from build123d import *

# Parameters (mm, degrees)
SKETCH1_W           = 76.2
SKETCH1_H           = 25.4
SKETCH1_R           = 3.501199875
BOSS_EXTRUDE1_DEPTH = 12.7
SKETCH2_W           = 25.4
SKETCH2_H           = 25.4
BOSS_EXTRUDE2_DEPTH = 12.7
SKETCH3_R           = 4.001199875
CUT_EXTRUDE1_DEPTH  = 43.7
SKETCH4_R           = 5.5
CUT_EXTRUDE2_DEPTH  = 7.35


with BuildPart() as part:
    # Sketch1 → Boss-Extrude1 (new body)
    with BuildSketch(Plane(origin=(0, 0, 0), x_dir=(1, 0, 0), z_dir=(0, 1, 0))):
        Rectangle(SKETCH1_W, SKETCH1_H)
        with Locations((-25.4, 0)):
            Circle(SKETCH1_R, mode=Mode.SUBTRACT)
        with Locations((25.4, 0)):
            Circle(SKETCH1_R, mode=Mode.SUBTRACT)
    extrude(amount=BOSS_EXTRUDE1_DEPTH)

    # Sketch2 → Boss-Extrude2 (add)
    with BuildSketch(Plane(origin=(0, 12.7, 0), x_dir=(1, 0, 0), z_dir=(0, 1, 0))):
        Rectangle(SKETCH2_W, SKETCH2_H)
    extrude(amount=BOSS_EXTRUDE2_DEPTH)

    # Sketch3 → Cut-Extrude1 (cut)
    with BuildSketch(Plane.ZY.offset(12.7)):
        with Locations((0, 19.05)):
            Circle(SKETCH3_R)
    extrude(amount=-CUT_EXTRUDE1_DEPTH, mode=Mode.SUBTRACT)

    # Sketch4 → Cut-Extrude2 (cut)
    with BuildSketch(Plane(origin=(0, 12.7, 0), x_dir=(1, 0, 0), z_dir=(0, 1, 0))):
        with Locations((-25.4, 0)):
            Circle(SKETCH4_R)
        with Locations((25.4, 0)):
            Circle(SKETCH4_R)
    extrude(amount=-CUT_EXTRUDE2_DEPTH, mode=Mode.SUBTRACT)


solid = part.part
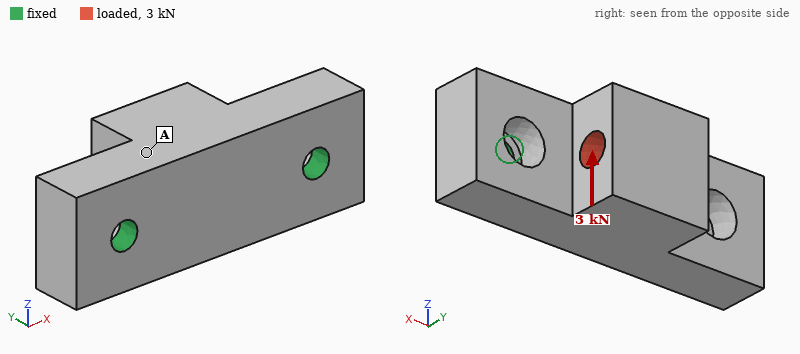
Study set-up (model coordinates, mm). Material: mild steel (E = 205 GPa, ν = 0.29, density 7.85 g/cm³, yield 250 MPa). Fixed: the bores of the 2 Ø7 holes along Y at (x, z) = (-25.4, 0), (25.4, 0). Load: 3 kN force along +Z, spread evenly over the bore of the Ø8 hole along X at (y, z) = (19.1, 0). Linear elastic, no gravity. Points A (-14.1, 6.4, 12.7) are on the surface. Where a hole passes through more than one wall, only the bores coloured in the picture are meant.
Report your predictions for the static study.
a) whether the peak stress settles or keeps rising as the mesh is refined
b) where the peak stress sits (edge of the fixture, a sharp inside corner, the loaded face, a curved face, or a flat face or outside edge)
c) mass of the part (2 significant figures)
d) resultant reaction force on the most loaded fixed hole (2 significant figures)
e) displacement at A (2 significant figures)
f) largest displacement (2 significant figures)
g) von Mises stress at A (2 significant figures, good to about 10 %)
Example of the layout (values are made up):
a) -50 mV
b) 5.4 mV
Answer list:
a) keeps rising
b) edge of the fixture
c) 230 g
d) 1.5 kN
e) 10 µm
f) 25 µm
g) 28 MPa
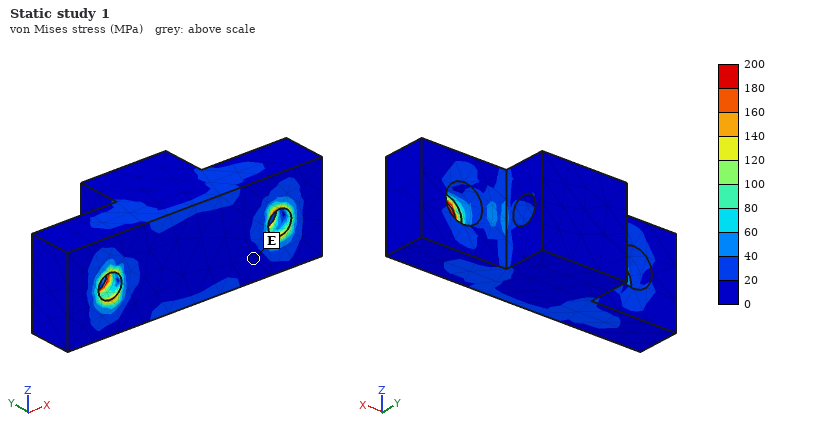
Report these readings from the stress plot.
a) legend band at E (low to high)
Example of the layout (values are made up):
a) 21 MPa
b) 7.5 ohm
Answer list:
a) 0 to 20 MPa
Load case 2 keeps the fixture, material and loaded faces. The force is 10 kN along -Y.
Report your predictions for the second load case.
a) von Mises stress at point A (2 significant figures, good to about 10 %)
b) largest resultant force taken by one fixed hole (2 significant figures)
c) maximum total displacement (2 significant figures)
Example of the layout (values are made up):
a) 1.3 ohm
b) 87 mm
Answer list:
a) 26 MPa
b) 6.2 kN
c) 13 µm
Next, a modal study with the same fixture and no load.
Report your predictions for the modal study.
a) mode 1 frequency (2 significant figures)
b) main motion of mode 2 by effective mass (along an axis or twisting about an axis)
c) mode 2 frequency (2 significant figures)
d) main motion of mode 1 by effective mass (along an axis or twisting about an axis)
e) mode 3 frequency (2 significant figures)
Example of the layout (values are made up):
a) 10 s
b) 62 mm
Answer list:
a) 6900 Hz
b) along Y
c) 13 kHz
d) along Z
e) 19 kHz
